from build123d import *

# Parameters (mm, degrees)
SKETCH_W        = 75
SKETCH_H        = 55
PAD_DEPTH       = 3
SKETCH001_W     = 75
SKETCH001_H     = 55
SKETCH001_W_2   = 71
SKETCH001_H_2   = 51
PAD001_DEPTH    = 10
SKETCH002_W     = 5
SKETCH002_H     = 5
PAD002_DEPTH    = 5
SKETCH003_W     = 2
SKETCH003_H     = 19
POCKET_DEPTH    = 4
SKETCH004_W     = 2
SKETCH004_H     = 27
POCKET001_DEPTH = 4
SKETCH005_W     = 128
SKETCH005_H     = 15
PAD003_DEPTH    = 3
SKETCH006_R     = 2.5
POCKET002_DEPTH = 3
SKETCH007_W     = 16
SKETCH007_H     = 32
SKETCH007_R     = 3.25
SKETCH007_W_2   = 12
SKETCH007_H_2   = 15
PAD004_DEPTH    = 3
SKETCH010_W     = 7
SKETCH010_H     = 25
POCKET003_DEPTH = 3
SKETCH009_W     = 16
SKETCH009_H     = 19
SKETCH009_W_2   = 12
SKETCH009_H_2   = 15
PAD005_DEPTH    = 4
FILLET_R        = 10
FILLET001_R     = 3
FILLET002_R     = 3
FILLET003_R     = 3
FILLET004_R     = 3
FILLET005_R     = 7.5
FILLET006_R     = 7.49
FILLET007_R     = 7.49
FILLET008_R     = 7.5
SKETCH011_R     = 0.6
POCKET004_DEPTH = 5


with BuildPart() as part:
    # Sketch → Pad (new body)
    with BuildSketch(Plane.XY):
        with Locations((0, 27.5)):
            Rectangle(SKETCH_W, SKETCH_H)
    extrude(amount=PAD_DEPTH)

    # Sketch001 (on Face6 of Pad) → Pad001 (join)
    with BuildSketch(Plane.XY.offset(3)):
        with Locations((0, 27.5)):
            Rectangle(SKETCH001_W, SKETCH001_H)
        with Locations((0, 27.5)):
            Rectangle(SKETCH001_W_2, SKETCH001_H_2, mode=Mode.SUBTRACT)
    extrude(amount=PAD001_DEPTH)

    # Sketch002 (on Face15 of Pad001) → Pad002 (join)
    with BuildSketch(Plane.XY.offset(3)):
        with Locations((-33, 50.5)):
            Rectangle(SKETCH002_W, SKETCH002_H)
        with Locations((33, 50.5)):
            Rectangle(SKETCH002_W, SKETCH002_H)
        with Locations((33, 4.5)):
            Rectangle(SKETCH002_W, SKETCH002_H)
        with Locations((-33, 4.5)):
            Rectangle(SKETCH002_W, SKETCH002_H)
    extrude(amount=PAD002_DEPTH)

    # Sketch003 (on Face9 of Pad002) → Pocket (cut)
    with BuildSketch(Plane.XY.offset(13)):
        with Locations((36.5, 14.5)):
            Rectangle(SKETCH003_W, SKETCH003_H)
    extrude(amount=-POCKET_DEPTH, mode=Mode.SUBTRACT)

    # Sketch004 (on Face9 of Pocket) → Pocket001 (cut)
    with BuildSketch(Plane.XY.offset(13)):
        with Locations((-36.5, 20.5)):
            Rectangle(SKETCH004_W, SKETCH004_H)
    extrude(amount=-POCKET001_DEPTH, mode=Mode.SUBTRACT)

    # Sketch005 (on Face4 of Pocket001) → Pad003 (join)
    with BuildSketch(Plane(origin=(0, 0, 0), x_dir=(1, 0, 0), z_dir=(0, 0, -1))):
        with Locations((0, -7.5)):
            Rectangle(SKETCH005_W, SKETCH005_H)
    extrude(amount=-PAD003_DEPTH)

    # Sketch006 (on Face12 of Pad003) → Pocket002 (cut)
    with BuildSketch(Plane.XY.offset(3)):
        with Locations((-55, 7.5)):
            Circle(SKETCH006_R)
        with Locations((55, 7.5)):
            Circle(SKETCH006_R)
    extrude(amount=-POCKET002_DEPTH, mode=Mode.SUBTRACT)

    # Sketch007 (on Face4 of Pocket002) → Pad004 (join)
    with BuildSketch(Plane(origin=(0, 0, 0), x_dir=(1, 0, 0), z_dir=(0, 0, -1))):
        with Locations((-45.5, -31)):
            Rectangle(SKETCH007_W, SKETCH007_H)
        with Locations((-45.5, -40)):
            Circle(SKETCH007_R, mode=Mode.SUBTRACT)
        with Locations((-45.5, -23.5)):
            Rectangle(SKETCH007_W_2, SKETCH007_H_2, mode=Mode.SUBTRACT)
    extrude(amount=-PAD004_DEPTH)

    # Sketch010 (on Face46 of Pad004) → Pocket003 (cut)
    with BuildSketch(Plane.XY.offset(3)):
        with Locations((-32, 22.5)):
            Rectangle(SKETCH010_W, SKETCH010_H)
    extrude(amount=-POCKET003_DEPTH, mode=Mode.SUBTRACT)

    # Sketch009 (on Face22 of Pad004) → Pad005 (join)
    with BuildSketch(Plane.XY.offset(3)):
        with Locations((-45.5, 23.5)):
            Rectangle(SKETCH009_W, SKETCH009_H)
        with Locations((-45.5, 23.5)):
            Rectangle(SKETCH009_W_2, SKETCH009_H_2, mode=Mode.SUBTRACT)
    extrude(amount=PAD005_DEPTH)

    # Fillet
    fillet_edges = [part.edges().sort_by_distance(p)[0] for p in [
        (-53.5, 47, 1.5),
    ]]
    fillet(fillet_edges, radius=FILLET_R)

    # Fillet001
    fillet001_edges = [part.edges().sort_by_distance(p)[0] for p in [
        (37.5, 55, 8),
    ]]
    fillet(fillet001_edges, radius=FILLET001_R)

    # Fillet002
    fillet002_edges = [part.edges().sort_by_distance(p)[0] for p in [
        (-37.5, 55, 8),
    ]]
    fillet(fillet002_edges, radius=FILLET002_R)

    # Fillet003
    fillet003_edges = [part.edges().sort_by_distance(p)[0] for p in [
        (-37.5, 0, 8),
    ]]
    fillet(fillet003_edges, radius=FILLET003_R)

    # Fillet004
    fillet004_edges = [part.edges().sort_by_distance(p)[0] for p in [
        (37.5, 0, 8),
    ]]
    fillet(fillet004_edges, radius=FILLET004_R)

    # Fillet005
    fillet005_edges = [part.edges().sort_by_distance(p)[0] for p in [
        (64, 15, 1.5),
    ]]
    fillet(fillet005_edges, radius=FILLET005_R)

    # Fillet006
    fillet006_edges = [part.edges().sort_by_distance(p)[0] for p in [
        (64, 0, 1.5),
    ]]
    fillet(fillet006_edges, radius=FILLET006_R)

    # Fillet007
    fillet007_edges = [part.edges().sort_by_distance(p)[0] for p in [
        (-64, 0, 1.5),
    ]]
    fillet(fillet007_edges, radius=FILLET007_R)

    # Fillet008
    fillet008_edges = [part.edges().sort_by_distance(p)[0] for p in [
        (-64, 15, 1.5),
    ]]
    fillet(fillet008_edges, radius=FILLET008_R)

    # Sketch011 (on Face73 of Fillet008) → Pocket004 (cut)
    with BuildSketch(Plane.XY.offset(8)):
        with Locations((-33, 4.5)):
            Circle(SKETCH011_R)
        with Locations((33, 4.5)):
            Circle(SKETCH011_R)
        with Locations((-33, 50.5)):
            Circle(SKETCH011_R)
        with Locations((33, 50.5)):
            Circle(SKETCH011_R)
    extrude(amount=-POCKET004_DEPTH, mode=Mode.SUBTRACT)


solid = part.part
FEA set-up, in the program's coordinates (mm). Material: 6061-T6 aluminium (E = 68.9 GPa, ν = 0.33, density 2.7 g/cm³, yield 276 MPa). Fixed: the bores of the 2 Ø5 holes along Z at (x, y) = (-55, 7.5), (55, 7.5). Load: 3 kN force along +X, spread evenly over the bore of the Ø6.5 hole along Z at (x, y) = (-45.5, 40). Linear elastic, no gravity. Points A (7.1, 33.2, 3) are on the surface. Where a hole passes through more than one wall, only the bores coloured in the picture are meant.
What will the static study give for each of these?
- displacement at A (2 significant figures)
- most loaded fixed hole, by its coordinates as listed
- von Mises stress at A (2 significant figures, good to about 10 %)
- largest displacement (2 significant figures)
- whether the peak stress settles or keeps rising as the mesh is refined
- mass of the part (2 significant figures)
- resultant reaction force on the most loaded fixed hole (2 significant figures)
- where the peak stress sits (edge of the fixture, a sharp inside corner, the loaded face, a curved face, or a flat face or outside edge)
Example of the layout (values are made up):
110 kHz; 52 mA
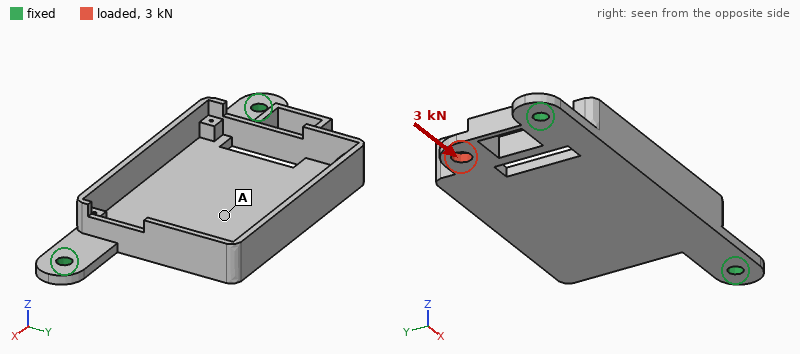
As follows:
0.055 mm; (55, 7.5); 23 MPa; 0.11 mm; keeps rising; 55 g; 2.0 kN; edge of the fixture
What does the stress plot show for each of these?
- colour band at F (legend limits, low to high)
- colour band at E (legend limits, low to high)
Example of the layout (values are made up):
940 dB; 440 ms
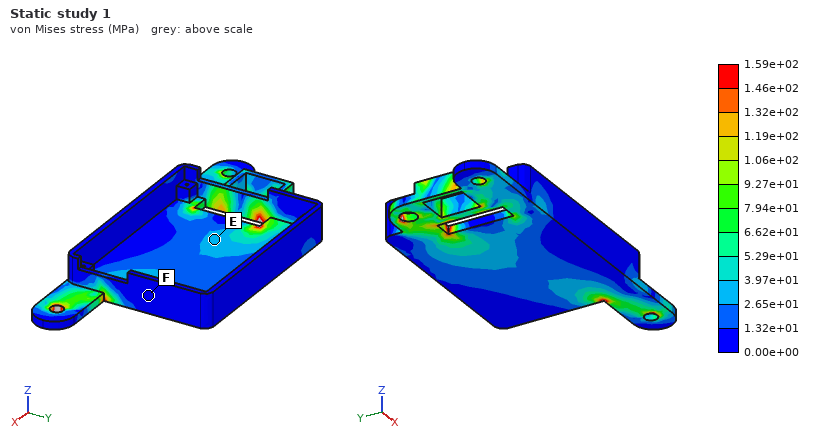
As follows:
0.00e+00 to 1.32e+01 MPa; 2.65e+01 to 3.97e+01 MPa
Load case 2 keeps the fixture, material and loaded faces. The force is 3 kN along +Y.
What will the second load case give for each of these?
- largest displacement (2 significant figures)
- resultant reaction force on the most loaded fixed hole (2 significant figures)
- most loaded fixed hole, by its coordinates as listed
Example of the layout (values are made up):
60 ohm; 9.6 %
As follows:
0.21 mm; 2.8 kN; (-55, 7.5)
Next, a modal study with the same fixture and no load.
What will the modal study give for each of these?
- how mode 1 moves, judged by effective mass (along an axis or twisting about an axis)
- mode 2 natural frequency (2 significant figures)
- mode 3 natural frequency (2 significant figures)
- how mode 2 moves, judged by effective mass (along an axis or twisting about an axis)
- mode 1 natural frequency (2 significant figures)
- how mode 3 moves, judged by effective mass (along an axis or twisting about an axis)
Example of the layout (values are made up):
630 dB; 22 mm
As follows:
along Z; 1500 Hz; 2300 Hz; twisting about Y; 560 Hz; along Z
